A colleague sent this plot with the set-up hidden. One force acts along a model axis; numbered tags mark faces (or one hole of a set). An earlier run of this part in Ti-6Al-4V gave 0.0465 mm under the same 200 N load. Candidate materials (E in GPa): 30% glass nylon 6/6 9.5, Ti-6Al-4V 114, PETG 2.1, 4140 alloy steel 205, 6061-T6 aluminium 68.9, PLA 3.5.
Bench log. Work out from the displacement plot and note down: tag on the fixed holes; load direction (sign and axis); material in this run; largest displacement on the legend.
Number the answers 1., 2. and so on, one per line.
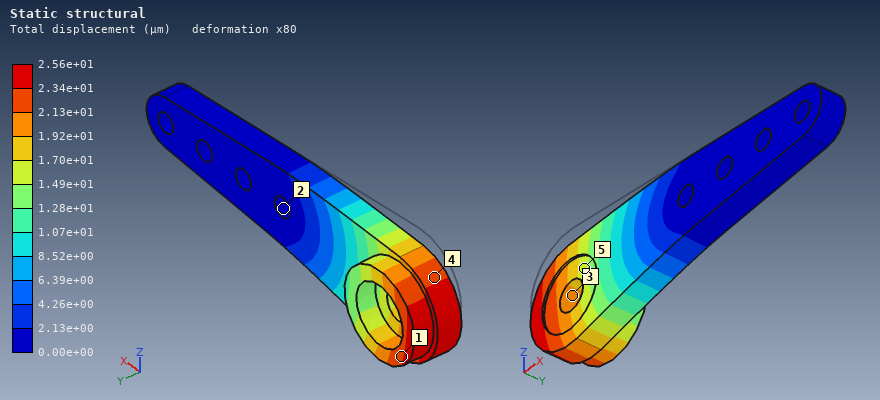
1. 2
2. -Z
3. 4140 alloy steel
4. 2.56e+01 µm
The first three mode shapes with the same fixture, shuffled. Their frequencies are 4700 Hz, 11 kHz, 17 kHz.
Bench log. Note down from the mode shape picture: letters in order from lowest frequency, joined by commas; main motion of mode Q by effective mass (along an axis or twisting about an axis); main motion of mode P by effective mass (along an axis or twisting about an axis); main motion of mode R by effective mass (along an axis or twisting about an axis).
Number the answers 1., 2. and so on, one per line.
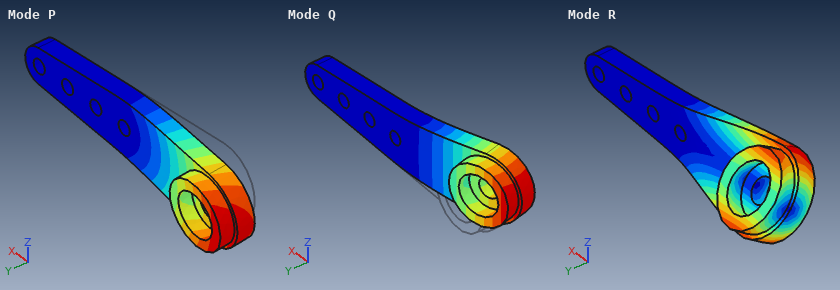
1. Q, P, R
2. along Y
3. along Z
4. twisting about X
